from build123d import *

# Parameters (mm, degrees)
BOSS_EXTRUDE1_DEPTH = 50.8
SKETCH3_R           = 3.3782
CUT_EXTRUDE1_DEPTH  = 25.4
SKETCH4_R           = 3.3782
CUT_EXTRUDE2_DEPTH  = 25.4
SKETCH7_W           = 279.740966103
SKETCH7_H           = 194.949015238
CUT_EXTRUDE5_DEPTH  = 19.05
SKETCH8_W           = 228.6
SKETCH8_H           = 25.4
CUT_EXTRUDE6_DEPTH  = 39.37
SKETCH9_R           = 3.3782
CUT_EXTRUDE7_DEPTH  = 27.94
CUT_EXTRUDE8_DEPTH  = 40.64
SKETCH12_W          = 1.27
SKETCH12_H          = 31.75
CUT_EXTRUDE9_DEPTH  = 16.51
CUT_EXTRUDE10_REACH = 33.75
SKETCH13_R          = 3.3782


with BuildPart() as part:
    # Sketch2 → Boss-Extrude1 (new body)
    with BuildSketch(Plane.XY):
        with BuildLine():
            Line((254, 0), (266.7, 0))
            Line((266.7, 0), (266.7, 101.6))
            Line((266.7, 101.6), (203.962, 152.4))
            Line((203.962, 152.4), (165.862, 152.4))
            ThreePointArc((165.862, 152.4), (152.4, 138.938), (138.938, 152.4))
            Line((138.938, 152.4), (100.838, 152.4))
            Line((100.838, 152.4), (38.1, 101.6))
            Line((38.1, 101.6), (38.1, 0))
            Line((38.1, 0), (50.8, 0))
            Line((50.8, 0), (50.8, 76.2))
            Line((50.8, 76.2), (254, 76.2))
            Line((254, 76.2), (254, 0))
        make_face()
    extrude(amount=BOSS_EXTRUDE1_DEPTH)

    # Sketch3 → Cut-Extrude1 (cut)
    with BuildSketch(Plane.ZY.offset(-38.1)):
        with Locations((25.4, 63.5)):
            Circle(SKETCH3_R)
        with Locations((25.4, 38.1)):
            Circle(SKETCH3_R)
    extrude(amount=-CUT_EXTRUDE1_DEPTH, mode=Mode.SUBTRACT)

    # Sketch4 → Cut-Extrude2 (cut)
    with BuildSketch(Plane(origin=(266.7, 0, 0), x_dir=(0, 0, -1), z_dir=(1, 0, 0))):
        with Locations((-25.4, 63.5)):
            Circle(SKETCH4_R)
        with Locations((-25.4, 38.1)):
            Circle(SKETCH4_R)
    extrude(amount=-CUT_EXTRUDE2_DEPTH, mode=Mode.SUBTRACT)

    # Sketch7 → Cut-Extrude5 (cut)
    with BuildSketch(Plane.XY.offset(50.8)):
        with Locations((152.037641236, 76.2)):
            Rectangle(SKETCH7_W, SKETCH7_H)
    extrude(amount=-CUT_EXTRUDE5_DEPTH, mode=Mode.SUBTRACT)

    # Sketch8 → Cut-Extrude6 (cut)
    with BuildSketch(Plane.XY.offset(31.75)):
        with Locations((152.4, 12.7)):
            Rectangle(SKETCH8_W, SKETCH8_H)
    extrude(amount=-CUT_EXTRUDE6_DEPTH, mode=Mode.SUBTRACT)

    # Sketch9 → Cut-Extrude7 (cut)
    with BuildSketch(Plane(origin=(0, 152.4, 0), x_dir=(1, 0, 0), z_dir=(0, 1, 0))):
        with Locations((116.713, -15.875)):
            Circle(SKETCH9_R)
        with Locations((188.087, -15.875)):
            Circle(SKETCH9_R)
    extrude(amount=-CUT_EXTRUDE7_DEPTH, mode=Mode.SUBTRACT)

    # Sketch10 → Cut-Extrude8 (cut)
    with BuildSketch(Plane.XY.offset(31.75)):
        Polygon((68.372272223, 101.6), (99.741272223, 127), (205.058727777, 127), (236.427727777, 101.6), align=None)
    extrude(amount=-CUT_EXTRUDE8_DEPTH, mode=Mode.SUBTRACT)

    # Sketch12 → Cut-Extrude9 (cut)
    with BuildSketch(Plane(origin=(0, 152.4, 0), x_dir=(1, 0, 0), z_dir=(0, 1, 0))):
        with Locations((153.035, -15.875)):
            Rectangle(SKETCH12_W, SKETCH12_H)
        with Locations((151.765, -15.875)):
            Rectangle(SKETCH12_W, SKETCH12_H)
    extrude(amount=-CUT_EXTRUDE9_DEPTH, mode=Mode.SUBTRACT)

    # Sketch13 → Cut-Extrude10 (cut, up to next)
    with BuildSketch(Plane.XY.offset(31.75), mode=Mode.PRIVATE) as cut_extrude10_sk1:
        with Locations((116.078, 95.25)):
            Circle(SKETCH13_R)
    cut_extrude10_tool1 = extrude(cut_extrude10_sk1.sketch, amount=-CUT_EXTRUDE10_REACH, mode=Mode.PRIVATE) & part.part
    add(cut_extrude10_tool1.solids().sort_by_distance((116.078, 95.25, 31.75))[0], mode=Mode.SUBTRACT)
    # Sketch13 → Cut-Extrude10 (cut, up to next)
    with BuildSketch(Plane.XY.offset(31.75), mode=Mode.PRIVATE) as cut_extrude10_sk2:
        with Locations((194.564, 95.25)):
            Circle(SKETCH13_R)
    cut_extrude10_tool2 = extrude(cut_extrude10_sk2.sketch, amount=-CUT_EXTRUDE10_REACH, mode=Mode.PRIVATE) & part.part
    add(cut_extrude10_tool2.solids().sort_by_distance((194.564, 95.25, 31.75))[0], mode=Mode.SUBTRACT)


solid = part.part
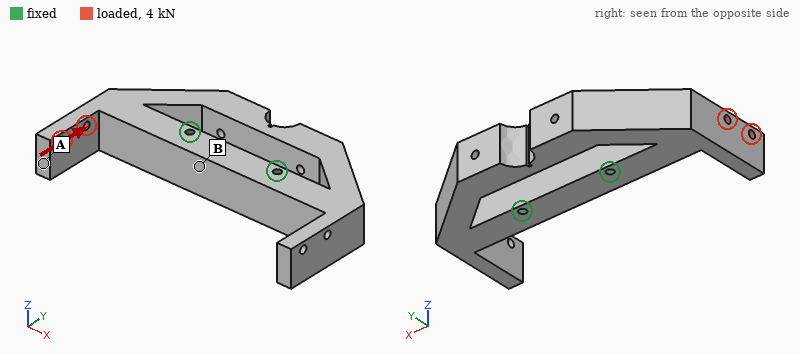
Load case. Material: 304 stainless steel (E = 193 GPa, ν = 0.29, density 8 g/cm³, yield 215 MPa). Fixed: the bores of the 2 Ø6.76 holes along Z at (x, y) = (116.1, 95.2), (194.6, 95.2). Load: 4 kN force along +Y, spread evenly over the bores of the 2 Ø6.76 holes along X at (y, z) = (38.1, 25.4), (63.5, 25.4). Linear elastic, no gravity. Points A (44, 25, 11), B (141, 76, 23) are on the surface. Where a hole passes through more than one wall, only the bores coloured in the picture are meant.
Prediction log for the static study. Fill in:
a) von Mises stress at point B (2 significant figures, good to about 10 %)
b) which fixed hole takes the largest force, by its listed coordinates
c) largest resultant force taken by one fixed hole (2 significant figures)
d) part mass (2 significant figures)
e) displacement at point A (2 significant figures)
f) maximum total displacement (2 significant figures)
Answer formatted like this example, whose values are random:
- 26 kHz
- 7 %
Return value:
- 19 MPa
- (116.1, 95.2)
- 6.4 kN
- 2.9 kg
- 83 µm
- 95 µm
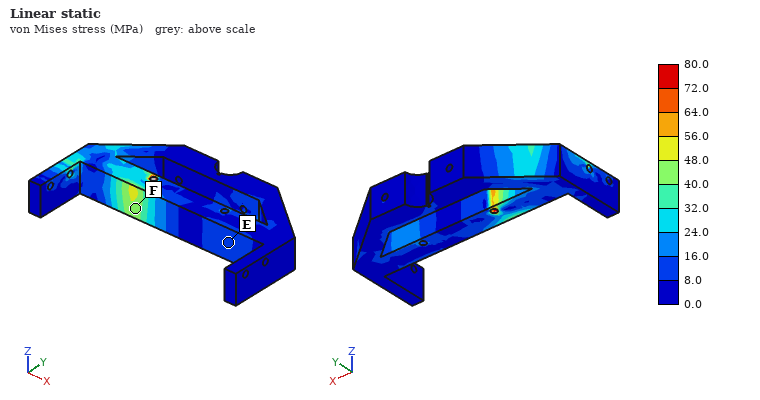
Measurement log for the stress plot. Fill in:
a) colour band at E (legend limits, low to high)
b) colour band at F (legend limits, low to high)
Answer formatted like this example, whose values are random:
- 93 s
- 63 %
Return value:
- 8.0 to 16.0 MPa
- 40.0 to 48.0 MPa
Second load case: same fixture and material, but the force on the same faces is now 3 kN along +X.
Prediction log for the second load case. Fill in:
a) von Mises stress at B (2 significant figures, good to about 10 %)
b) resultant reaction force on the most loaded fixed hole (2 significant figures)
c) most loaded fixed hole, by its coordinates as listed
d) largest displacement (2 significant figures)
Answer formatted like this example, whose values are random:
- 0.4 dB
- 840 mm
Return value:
- 8.3 MPa
- 3.0 kN
- (116.1, 95.2)
- 0.14 mm
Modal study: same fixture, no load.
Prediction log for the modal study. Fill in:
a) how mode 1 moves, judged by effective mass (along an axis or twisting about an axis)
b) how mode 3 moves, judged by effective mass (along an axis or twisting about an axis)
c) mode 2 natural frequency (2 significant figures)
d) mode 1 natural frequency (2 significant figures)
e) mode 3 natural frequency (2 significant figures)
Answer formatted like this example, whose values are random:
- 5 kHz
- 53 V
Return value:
- along Z
- along Y
- 1400 Hz
- 1300 Hz
- 1700 Hz
